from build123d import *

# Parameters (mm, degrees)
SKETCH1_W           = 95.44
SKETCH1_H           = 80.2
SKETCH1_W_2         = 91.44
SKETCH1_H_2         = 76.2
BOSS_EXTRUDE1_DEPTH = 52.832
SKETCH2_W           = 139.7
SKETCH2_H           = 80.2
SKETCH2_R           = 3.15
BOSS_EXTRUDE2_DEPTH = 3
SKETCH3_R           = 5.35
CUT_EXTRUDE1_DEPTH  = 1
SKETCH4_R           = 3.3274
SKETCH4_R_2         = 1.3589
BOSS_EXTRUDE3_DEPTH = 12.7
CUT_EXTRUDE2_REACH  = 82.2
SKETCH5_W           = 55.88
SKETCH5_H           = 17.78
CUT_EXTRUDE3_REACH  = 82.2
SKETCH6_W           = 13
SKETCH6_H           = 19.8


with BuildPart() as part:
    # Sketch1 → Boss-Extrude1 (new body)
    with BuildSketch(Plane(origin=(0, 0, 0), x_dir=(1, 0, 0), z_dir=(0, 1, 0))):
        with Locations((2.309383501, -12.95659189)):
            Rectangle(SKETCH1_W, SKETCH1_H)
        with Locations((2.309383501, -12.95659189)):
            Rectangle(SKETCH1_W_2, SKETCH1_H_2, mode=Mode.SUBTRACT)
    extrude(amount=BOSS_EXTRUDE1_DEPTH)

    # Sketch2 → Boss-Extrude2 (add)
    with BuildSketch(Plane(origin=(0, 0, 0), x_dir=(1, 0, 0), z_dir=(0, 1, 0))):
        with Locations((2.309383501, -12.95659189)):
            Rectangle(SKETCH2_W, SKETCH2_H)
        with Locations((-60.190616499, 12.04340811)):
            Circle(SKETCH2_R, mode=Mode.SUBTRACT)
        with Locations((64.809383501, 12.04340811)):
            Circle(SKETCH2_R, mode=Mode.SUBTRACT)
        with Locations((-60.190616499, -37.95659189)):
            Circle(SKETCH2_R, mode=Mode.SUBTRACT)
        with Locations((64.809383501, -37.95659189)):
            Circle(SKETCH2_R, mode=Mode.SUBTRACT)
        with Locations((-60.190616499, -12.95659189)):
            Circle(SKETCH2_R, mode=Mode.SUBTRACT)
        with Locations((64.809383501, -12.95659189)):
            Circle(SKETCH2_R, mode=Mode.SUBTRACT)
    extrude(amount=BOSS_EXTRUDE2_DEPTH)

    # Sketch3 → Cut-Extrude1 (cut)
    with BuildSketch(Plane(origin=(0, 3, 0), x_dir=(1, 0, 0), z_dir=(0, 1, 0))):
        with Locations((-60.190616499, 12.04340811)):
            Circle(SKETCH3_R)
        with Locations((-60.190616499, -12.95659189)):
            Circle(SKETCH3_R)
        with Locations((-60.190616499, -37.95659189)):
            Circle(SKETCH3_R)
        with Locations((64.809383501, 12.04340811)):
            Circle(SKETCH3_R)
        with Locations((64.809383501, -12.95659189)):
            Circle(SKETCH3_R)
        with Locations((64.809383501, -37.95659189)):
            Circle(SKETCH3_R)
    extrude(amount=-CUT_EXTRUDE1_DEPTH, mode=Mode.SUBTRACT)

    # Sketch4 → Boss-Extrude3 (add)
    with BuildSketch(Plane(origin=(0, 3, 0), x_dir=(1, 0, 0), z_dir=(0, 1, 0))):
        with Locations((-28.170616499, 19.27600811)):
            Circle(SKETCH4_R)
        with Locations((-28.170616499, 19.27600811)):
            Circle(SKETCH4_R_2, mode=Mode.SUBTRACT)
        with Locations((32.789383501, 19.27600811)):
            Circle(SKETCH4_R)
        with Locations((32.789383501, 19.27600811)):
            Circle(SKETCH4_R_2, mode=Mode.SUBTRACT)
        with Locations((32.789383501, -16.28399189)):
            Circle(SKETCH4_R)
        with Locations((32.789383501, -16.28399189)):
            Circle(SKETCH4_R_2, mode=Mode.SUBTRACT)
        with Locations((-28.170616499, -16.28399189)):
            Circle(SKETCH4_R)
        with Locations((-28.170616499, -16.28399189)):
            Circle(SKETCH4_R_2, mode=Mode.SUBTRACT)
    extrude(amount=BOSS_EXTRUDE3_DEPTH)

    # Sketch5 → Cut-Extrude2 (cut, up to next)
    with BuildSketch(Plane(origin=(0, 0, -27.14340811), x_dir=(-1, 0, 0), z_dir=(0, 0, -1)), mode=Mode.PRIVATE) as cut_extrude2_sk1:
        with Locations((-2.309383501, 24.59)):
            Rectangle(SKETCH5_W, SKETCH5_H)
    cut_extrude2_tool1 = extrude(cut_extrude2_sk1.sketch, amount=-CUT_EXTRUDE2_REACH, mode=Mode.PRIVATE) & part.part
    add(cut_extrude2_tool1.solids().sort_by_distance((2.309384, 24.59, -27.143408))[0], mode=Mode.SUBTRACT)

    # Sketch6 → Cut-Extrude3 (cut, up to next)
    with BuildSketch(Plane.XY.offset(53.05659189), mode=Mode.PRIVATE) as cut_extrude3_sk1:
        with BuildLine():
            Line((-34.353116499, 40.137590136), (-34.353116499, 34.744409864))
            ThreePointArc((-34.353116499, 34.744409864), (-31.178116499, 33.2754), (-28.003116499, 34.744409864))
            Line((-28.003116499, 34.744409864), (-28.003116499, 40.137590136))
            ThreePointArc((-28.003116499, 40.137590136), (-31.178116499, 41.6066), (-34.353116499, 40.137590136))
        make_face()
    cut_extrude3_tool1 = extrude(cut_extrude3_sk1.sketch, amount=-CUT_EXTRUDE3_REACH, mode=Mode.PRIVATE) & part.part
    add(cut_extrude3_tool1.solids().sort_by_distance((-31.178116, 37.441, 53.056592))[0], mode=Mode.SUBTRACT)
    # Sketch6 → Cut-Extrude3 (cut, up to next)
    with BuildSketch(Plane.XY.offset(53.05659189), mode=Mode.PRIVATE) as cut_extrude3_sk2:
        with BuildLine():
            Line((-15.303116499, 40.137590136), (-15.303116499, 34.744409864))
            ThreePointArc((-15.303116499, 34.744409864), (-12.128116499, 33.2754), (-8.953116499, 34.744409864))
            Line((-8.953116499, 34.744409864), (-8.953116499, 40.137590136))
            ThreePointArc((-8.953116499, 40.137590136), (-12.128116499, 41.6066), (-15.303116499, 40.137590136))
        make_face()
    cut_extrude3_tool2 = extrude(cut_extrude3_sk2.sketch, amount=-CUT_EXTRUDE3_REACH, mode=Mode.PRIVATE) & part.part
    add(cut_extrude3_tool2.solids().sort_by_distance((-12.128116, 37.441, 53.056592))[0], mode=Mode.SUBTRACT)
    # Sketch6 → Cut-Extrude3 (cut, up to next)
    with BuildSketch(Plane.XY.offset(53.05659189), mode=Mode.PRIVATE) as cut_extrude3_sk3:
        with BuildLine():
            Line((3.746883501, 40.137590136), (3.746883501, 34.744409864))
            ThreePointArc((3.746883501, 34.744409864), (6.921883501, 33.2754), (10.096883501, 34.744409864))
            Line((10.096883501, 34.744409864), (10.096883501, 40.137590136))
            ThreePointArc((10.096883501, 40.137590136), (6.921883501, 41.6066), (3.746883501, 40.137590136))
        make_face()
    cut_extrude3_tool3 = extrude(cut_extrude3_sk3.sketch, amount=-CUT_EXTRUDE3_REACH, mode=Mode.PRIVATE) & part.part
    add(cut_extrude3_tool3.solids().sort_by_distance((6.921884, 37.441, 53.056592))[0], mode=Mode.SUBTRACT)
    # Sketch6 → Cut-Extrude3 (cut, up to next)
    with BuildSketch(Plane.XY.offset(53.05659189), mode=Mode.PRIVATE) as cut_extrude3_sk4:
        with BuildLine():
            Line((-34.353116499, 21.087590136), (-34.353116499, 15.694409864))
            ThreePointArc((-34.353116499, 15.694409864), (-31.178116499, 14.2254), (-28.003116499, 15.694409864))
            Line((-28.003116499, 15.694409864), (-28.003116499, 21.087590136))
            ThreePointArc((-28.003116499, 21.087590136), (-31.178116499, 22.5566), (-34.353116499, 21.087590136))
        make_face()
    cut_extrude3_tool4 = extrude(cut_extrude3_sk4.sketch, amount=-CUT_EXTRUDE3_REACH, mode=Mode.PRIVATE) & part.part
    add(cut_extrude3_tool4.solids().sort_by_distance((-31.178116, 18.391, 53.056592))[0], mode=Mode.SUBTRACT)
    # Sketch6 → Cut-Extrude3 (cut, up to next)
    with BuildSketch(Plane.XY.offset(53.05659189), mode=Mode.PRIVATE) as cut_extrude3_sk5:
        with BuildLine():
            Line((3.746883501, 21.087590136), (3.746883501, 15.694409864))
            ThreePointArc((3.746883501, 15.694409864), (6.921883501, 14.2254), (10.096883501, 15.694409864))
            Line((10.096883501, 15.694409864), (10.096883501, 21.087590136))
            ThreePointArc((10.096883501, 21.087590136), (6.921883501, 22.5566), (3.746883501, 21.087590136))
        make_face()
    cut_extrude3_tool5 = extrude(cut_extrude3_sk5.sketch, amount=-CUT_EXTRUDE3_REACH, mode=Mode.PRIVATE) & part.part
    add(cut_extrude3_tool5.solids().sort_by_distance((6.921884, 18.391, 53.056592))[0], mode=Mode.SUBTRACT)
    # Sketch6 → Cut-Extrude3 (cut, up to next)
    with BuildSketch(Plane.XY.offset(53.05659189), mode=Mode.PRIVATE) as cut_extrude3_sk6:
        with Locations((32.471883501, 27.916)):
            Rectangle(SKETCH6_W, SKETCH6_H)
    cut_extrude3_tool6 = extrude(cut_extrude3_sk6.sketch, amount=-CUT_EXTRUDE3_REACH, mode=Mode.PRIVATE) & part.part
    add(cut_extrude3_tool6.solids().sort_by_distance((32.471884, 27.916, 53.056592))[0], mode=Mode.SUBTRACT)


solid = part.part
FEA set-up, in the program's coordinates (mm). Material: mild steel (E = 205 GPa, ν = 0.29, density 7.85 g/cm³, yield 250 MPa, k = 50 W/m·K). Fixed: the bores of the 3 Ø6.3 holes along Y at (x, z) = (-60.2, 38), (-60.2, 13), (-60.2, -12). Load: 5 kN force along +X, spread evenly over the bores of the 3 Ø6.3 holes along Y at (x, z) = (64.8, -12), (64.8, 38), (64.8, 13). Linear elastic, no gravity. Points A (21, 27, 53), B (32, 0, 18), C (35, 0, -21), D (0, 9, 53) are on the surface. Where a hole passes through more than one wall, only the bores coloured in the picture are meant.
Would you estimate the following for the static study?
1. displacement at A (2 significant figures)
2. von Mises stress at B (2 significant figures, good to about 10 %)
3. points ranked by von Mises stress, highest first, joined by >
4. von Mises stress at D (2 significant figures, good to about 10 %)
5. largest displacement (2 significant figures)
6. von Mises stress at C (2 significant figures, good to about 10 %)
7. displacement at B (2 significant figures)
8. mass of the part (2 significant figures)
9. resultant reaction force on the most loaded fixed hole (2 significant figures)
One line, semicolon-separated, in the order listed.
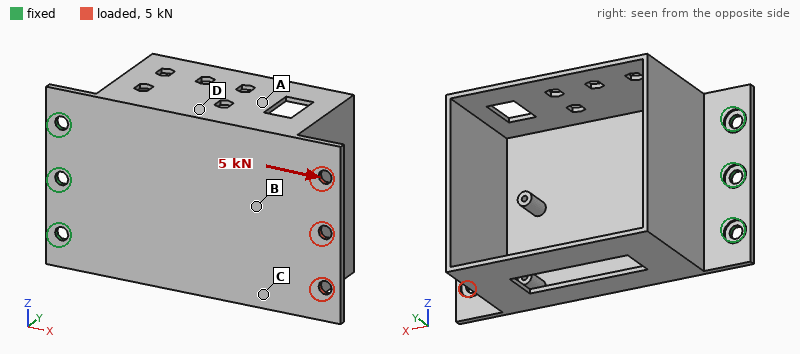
0.090 mm; 27 MPa; B > C > D > A; 12 MPa; 0.19 mm; 19 MPa; 0.098 mm; 510 g; 1.8 kN
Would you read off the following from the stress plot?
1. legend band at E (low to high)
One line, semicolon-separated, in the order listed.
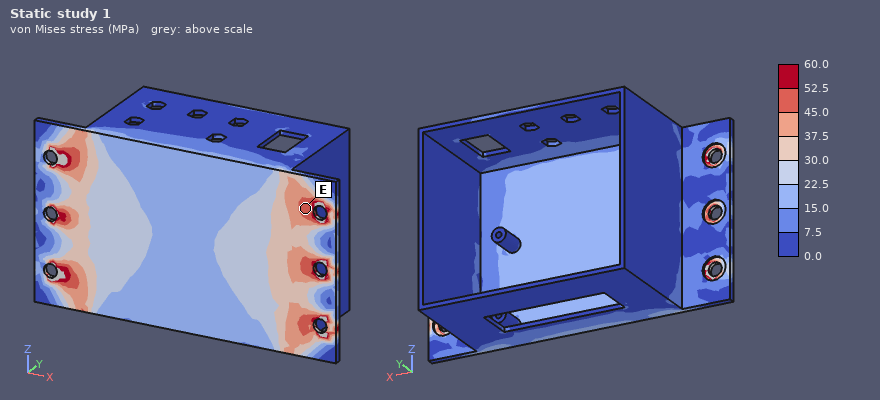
45.0 to 52.5 MPa
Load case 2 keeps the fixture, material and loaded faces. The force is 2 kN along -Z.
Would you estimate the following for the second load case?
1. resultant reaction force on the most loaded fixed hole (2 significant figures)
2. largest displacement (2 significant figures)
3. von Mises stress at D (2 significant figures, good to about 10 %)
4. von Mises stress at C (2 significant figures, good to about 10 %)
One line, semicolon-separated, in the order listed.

4.7 kN; 0.11 mm; 21 MPa; 16 MPa
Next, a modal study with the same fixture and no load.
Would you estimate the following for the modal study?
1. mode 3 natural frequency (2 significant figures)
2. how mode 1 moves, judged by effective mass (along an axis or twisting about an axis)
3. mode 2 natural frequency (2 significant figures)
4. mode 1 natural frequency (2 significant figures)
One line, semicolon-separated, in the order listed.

1100 Hz; along Y; 350 Hz; 130 Hz
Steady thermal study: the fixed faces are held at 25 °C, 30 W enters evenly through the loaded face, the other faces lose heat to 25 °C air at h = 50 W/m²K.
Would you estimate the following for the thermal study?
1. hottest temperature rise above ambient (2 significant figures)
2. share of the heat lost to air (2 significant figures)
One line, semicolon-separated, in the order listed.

79 K; 98 %
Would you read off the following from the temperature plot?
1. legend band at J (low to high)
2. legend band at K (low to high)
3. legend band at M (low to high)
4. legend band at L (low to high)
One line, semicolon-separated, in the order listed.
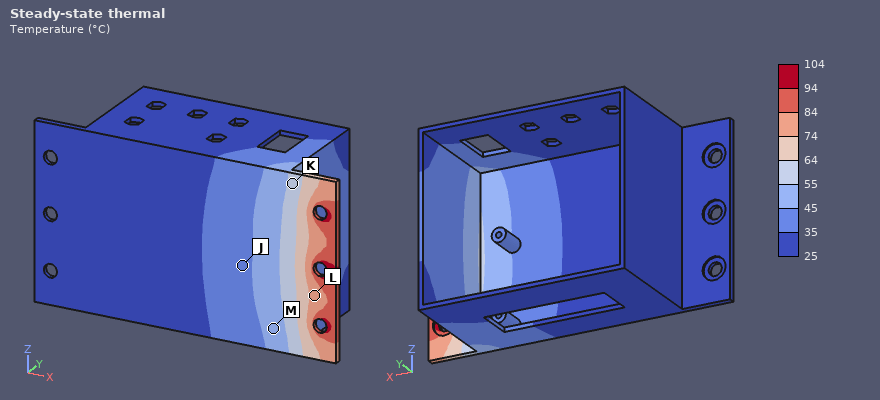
35 to 45 °C; 55 to 64 °C; 45 to 55 °C; 74 to 84 °C
